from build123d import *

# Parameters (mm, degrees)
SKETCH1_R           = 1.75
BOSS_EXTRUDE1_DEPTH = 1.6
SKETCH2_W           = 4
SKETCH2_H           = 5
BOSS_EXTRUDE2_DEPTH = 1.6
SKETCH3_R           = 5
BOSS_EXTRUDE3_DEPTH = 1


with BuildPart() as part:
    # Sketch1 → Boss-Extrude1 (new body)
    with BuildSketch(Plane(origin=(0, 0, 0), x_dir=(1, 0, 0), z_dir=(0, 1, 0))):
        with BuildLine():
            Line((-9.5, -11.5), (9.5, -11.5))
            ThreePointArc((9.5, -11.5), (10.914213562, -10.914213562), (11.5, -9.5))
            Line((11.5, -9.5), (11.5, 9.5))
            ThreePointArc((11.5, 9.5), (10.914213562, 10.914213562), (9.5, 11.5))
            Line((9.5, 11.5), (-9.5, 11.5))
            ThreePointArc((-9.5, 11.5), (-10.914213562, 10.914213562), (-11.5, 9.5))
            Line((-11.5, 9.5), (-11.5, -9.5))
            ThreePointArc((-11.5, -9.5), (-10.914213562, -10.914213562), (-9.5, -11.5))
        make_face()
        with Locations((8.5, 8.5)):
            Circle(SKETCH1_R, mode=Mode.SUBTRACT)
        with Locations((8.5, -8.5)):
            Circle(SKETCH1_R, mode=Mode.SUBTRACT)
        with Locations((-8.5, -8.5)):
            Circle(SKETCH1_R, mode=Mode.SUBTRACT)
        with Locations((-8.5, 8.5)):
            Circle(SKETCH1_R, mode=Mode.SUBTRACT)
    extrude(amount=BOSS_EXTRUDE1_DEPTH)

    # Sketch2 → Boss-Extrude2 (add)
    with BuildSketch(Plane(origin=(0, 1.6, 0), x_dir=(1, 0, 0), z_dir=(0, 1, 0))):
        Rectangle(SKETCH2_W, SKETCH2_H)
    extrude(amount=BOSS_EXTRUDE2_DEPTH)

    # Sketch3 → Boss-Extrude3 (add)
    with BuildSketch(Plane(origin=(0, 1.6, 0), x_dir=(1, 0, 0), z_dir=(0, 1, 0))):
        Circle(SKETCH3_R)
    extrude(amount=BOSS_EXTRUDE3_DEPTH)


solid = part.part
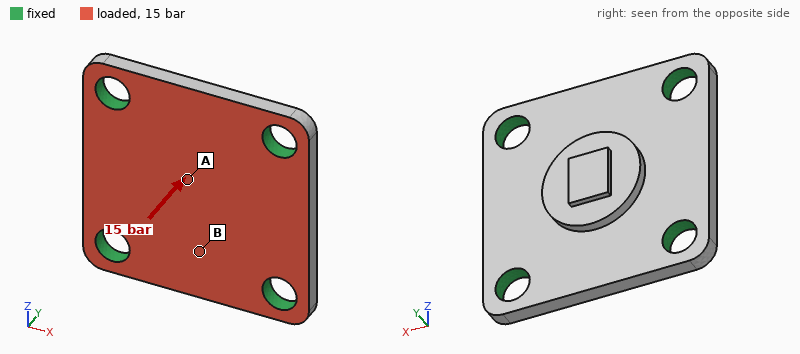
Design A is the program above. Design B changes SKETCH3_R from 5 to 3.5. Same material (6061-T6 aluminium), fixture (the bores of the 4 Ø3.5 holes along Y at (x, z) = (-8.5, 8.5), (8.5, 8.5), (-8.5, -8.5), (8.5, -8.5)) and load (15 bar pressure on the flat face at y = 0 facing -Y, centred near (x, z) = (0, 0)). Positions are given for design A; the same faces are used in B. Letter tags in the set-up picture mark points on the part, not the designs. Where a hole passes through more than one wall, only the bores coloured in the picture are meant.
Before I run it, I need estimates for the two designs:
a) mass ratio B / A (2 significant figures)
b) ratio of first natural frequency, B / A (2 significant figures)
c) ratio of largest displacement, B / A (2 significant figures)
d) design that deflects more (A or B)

0.95
0.96
1.2
B
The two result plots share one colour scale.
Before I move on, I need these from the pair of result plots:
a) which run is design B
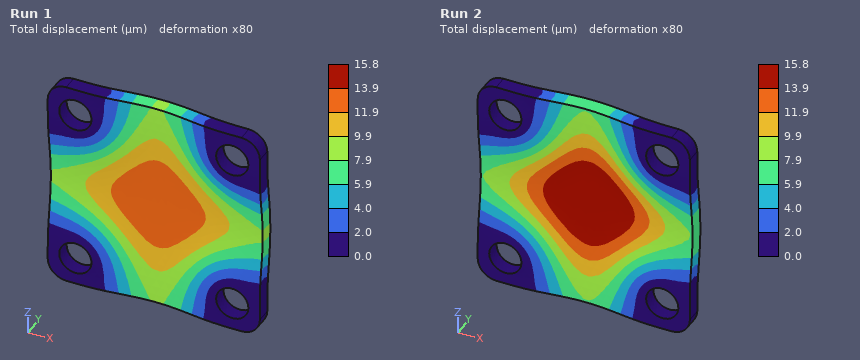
Run 2
